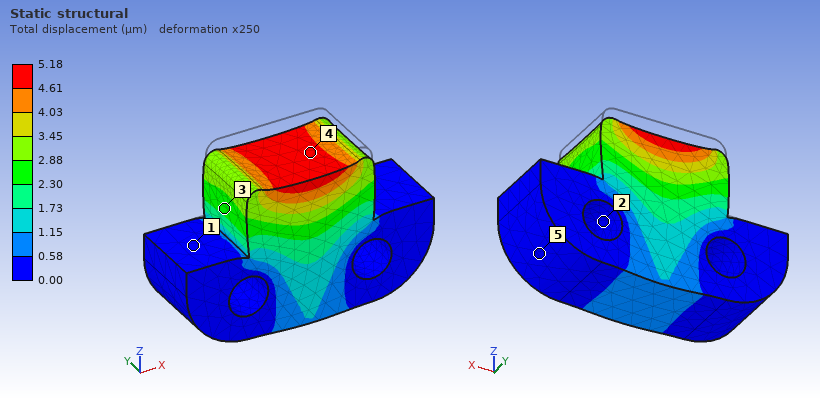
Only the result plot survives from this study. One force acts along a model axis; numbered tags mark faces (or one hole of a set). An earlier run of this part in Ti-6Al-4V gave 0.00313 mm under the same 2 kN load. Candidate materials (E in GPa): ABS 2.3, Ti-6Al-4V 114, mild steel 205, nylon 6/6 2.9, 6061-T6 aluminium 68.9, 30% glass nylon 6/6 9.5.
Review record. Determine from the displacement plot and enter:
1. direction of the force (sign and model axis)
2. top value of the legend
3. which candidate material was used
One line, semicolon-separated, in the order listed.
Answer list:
-Z; 5.18 µm; 6061-T6 aluminium
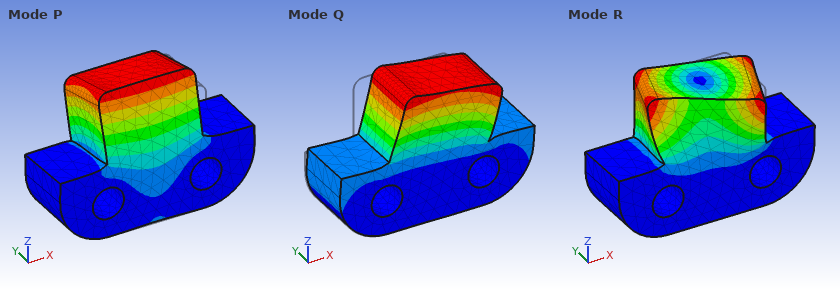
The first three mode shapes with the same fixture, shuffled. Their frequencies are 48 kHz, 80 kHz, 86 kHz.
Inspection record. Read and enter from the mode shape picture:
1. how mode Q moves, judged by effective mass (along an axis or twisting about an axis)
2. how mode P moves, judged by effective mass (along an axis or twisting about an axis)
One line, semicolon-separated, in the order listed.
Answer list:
along X; along Y
